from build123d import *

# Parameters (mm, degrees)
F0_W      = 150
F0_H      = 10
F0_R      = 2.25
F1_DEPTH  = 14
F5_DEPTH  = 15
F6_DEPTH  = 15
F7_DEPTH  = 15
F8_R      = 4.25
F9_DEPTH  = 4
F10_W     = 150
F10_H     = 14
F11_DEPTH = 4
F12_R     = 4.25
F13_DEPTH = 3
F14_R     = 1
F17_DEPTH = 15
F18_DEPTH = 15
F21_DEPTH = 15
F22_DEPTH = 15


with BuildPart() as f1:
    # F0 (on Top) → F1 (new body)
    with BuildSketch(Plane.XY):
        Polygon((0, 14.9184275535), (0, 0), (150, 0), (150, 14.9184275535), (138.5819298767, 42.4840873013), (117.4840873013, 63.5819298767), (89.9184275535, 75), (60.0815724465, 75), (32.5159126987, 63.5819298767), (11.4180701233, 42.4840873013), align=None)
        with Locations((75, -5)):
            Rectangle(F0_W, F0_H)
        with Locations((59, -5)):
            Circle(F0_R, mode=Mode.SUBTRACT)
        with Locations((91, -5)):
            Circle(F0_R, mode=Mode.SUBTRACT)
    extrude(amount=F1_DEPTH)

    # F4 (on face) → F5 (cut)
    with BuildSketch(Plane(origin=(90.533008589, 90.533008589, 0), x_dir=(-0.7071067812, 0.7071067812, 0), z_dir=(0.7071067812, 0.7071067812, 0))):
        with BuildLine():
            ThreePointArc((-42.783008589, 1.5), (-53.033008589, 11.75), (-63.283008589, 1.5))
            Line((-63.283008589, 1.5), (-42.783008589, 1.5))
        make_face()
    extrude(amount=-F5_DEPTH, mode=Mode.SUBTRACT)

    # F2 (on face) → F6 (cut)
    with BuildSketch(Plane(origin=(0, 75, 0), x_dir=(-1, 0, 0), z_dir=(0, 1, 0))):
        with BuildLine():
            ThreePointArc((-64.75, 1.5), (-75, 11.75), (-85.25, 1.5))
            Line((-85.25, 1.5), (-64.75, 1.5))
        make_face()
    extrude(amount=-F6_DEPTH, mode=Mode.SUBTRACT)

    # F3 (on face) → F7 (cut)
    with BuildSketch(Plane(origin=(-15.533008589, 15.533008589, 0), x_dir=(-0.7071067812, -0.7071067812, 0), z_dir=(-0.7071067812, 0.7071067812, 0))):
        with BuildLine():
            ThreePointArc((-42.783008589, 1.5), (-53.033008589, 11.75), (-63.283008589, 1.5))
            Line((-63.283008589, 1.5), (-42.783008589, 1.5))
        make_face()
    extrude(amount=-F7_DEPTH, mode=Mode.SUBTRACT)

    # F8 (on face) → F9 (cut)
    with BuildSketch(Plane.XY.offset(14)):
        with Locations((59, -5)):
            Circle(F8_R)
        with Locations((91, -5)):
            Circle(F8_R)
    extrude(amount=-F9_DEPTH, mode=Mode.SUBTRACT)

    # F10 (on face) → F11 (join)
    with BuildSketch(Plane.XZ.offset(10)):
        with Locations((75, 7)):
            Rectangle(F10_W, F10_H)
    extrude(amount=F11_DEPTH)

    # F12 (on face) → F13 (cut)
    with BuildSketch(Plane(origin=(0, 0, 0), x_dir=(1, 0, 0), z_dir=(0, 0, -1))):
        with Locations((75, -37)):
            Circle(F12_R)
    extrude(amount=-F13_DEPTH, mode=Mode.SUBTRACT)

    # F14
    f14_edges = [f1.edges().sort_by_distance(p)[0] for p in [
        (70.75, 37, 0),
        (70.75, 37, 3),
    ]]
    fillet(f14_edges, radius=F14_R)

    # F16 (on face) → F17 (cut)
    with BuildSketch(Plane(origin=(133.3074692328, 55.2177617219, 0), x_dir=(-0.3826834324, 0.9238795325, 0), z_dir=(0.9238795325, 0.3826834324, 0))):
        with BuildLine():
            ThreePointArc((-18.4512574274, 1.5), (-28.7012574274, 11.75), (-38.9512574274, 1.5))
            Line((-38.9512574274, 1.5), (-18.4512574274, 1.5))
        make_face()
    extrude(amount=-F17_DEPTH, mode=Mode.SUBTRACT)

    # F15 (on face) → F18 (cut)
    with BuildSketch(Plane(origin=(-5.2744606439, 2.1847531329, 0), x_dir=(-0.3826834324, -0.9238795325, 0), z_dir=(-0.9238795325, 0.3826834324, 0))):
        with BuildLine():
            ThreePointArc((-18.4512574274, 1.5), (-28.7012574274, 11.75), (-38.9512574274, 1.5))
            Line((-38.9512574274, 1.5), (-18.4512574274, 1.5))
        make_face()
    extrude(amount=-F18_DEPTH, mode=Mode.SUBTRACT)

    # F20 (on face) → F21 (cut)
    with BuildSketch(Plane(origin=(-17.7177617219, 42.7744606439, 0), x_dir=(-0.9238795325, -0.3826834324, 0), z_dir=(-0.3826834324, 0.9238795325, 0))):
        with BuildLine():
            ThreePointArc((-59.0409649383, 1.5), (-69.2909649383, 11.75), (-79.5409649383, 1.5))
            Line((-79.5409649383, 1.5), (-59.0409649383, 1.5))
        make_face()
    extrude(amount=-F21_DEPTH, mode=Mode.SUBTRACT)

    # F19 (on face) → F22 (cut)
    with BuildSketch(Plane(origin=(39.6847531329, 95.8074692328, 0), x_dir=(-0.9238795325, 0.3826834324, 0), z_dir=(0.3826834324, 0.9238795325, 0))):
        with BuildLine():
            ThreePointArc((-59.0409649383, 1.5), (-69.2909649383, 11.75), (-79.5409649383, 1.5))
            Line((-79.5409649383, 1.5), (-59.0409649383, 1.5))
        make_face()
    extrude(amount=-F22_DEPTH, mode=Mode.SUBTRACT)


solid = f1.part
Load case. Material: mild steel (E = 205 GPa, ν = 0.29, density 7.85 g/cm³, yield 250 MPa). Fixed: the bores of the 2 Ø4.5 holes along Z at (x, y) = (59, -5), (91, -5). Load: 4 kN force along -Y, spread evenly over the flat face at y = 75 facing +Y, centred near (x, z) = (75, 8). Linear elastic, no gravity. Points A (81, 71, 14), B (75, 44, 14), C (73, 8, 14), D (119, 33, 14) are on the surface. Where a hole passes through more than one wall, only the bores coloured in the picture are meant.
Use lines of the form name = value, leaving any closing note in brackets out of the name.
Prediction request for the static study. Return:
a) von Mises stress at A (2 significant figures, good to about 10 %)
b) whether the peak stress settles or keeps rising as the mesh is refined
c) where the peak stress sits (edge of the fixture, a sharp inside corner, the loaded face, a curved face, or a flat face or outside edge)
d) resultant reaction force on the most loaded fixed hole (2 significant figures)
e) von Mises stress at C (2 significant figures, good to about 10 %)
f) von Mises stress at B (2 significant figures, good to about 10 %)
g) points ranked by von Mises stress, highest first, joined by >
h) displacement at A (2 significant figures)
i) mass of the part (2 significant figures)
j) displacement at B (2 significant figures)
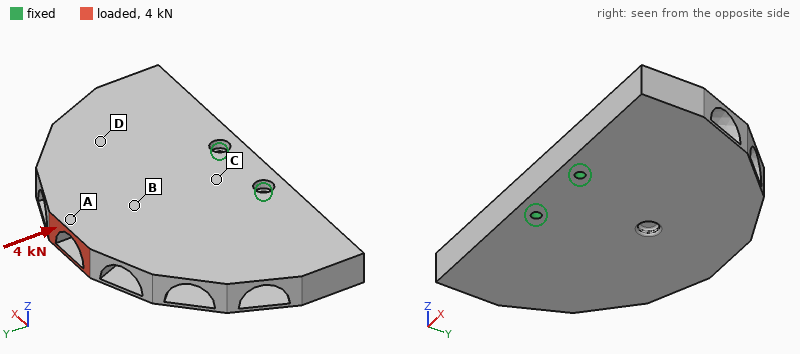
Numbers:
von Mises stress at A = 14 MPa
whether the peak stress settles or keeps rising as the mesh is refined = keeps rising
where the peak stress sits = edge of the fixture
resultant reaction force on the most loaded fixed hole = 2.0 kN
von Mises stress at C = 4.9 MPa
von Mises stress at B = 7.5 MPa
points ranked by von Mises stress, highest first, joined by > = A > B > C > D
displacement at A = 8.1 µm
mass of the part = 1.1 kg
displacement at B = 4.8 µm
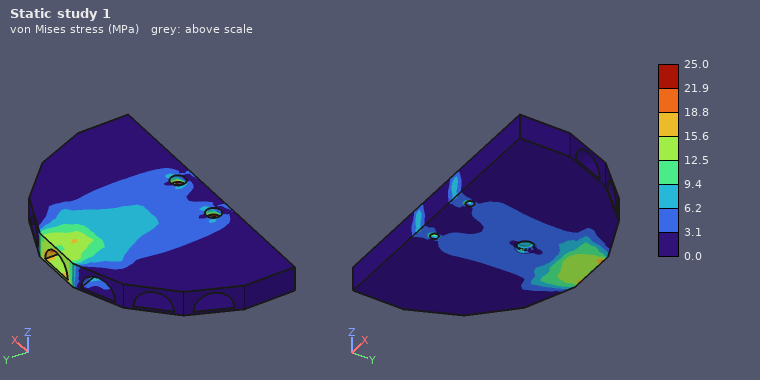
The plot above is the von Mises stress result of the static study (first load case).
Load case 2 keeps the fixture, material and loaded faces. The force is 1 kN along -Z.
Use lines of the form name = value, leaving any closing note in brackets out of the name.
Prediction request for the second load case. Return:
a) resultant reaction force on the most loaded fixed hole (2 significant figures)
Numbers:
resultant reaction force on the most loaded fixed hole = 540 N
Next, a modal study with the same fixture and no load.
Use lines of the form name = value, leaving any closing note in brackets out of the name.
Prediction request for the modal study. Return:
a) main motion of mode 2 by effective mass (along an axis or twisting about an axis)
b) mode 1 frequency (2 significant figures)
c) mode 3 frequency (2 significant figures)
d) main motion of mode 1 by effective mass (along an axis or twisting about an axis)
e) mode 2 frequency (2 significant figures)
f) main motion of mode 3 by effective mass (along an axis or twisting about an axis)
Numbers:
main motion of mode 2 by effective mass = twisting about Y
mode 1 frequency = 1400 Hz
mode 3 frequency = 3000 Hz
main motion of mode 1 by effective mass = along Z
mode 2 frequency = 2100 Hz
main motion of mode 3 by effective mass = along Z
